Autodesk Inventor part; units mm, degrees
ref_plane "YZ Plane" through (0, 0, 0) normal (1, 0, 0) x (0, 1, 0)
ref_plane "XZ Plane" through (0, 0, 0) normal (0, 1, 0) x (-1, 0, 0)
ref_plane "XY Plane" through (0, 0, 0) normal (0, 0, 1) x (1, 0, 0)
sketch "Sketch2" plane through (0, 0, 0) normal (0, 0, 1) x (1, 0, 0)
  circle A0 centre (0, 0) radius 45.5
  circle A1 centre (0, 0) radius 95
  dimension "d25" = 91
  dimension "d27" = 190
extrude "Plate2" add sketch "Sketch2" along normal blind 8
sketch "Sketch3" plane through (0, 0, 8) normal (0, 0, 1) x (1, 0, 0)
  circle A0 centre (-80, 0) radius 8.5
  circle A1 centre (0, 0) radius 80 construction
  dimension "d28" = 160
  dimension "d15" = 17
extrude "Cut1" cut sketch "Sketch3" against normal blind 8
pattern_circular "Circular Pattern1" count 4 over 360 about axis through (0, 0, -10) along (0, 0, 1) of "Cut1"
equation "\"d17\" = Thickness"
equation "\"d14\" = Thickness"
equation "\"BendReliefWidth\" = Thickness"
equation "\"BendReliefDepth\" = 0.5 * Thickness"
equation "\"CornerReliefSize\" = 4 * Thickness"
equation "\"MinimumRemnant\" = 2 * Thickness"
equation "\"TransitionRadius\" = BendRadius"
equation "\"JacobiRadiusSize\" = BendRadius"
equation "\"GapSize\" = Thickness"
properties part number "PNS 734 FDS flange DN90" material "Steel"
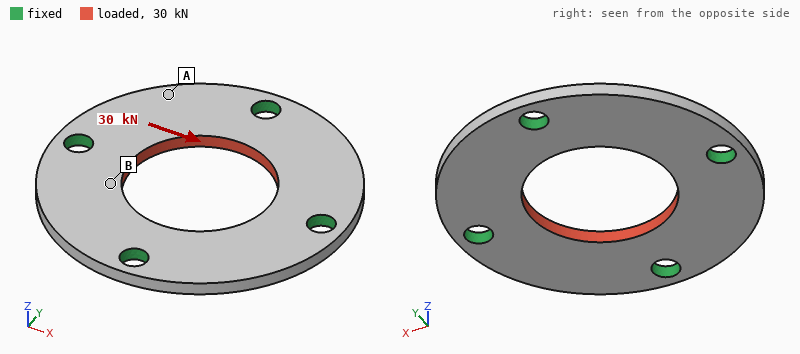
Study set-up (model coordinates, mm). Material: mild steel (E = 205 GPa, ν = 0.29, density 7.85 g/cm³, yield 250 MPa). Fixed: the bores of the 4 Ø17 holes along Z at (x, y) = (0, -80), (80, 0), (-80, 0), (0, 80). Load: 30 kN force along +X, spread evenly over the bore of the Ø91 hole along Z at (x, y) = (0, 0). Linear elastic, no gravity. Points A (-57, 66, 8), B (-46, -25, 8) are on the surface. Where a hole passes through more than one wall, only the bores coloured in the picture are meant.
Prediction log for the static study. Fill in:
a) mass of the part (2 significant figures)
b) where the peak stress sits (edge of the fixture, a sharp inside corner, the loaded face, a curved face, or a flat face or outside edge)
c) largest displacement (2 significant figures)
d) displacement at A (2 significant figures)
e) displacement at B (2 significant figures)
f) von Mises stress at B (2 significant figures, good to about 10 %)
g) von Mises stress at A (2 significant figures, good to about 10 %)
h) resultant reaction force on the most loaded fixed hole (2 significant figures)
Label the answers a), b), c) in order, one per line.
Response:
a) 1.3 kg
b) edge of the fixture
c) 6.5 µm
d) 4.4 µm
e) 4.9 µm
f) 18 MPa
g) 11 MPa
h) 7.7 kN
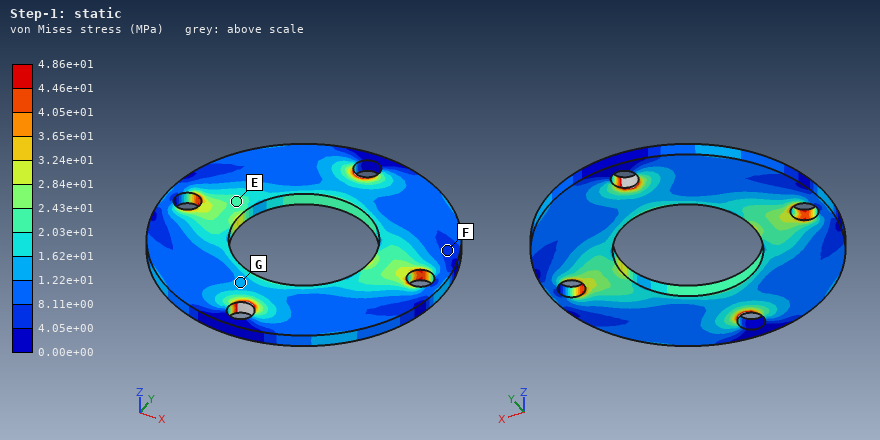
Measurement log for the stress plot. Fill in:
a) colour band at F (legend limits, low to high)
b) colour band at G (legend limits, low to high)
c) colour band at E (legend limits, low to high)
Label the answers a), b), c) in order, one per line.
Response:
a) 4.05e+00 to 8.11e+00 MPa
b) 1.22e+01 to 1.62e+01 MPa
c) 2.03e+01 to 2.43e+01 MPa
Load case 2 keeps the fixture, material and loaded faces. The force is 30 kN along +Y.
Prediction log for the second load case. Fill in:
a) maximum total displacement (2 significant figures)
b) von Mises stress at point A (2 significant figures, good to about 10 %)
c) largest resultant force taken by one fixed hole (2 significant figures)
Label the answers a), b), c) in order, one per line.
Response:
a) 6.5 µm
b) 9.7 MPa
c) 7.7 kN
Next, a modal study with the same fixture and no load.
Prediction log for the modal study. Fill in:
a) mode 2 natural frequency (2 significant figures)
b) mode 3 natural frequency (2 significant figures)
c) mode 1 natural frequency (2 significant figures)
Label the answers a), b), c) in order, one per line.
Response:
a) 3100 Hz
b) 3100 Hz
c) 3000 Hz
